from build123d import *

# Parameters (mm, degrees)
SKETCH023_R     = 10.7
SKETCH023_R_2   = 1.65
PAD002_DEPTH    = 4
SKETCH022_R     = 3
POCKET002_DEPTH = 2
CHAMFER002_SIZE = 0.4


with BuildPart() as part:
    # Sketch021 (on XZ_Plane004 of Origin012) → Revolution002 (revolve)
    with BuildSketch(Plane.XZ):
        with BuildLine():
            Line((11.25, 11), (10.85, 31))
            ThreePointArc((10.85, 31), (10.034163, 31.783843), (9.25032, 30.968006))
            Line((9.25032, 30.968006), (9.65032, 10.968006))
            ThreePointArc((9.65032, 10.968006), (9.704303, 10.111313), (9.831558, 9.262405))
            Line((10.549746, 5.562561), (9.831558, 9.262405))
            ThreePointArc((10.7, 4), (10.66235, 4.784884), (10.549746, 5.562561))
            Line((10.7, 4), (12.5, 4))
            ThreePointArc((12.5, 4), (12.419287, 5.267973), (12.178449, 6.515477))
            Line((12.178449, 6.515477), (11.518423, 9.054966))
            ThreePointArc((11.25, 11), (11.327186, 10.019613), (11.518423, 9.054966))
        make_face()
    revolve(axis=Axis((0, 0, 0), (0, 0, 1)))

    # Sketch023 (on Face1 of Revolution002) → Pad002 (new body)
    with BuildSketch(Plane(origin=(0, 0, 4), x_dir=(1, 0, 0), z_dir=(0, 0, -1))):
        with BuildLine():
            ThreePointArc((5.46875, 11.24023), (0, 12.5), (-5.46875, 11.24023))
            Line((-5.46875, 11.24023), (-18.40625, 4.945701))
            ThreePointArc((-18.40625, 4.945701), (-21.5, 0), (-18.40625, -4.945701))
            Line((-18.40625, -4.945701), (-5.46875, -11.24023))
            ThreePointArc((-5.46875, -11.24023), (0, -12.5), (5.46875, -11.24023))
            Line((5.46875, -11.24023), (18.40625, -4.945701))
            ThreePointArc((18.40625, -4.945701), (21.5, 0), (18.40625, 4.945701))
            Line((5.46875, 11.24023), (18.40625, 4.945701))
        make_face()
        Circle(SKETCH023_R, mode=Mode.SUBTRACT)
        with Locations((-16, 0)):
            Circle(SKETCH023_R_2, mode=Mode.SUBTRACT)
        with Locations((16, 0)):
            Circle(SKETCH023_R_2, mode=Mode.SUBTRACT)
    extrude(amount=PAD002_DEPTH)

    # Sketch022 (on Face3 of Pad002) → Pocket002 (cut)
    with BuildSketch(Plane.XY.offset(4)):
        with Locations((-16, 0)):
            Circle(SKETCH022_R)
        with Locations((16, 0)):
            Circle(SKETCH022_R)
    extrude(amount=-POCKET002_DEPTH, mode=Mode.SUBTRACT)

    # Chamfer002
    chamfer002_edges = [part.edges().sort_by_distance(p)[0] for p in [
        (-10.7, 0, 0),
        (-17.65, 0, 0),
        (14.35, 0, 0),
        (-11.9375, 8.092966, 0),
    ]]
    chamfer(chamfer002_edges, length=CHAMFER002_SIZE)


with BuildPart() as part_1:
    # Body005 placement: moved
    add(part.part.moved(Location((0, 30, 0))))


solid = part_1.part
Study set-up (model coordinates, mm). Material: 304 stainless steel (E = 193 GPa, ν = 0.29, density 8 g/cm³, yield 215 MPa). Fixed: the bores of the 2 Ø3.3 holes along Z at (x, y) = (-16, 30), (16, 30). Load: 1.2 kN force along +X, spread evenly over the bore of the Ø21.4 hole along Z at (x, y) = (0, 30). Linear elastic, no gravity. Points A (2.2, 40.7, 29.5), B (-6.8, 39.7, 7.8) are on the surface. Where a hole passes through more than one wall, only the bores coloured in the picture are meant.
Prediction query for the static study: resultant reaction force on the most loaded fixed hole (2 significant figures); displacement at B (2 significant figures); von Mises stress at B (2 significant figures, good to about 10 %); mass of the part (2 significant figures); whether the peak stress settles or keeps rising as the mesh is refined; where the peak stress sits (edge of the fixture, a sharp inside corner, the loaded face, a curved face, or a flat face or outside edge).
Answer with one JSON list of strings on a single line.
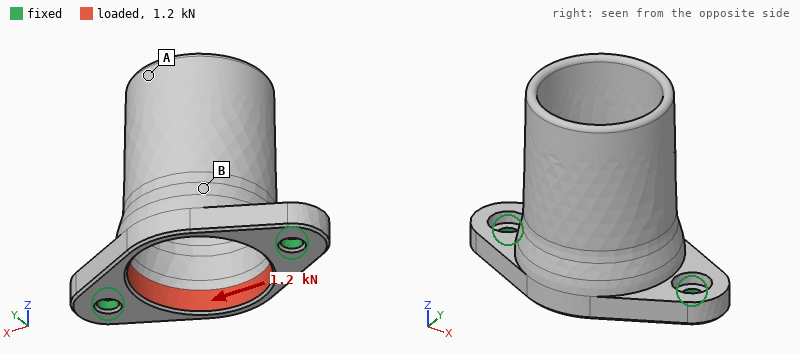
["600 N", "2.7 µm", "11 MPa", "34 g", "keeps rising", "edge of the fixture"]
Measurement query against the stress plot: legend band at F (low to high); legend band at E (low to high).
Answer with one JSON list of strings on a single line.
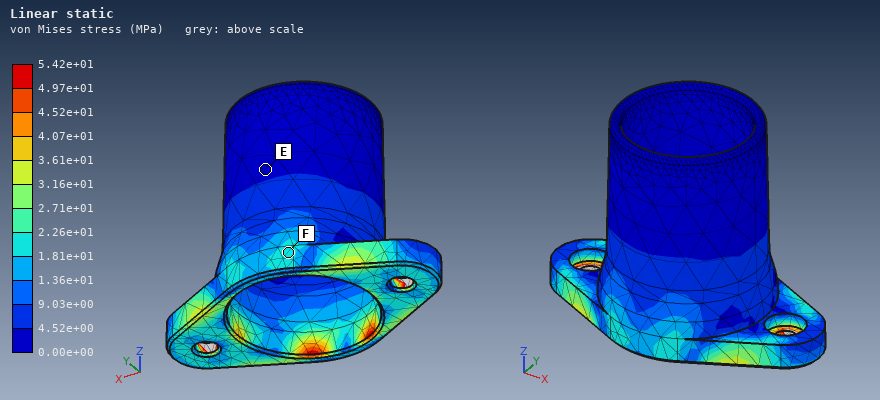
["1.81e+01 to 2.26e+01 MPa", "0.00e+00 to 4.52e+00 MPa"]
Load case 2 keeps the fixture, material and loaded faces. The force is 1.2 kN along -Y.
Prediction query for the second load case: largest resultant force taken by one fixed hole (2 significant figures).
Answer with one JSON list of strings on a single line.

["600 N"]
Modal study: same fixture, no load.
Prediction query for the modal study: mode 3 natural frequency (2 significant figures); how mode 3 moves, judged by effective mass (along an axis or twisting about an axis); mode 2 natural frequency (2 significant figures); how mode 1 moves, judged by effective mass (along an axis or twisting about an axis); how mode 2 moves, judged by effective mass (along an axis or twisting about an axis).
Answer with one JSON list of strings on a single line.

["11 kHz", "along X", "9400 Hz", "along Y", "along Z"]
